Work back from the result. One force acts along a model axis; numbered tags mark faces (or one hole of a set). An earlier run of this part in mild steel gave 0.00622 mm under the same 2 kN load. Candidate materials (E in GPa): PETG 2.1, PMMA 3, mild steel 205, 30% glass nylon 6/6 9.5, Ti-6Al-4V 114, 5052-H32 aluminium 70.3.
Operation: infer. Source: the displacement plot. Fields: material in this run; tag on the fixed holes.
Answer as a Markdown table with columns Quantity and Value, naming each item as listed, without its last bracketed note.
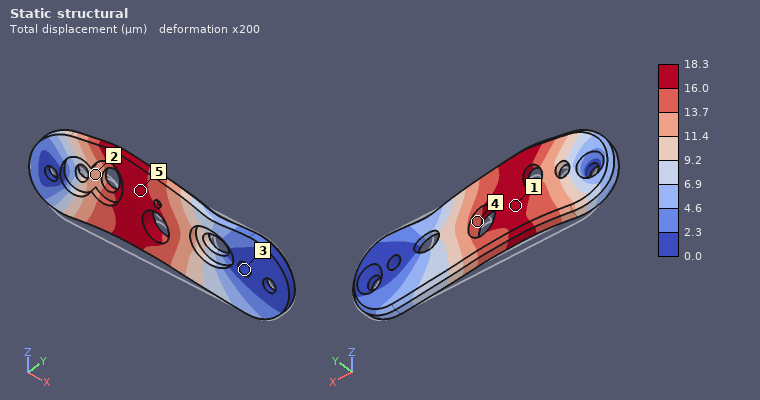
| Quantity | Value |
|---|---|
| material in this run | 5052-H32 aluminium |
| tag on the fixed holes | 3 |
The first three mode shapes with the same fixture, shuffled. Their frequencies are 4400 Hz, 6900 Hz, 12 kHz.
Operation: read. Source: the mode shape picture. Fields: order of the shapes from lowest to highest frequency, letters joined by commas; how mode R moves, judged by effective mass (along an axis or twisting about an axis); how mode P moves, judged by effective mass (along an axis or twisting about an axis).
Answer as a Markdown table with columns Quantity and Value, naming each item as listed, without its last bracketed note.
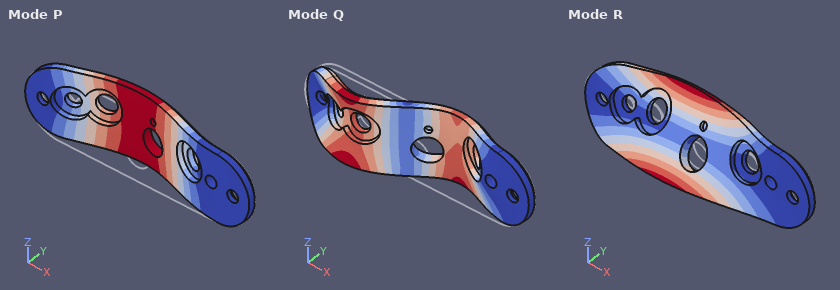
| Quantity | Value |
|---|---|
| order of the shapes from lowest to highest frequency, letters joined by commas | P, R, Q |
| how mode R moves, judged by effective mass | twisting about X |
| how mode P moves, judged by effective mass | along Y |
